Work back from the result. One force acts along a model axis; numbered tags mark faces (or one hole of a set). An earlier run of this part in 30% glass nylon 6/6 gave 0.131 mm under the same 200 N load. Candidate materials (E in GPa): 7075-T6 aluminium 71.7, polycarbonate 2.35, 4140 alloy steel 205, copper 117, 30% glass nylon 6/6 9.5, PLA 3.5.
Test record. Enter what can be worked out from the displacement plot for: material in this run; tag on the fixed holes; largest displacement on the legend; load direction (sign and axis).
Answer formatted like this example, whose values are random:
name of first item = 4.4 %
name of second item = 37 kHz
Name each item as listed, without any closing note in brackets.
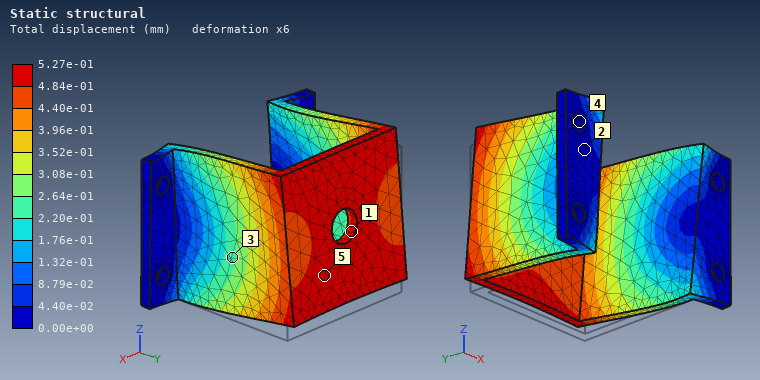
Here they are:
material in this run = polycarbonate
tag on the fixed holes = 4
largest displacement on the legend = 5.27e-01 mm
load direction = +Z
